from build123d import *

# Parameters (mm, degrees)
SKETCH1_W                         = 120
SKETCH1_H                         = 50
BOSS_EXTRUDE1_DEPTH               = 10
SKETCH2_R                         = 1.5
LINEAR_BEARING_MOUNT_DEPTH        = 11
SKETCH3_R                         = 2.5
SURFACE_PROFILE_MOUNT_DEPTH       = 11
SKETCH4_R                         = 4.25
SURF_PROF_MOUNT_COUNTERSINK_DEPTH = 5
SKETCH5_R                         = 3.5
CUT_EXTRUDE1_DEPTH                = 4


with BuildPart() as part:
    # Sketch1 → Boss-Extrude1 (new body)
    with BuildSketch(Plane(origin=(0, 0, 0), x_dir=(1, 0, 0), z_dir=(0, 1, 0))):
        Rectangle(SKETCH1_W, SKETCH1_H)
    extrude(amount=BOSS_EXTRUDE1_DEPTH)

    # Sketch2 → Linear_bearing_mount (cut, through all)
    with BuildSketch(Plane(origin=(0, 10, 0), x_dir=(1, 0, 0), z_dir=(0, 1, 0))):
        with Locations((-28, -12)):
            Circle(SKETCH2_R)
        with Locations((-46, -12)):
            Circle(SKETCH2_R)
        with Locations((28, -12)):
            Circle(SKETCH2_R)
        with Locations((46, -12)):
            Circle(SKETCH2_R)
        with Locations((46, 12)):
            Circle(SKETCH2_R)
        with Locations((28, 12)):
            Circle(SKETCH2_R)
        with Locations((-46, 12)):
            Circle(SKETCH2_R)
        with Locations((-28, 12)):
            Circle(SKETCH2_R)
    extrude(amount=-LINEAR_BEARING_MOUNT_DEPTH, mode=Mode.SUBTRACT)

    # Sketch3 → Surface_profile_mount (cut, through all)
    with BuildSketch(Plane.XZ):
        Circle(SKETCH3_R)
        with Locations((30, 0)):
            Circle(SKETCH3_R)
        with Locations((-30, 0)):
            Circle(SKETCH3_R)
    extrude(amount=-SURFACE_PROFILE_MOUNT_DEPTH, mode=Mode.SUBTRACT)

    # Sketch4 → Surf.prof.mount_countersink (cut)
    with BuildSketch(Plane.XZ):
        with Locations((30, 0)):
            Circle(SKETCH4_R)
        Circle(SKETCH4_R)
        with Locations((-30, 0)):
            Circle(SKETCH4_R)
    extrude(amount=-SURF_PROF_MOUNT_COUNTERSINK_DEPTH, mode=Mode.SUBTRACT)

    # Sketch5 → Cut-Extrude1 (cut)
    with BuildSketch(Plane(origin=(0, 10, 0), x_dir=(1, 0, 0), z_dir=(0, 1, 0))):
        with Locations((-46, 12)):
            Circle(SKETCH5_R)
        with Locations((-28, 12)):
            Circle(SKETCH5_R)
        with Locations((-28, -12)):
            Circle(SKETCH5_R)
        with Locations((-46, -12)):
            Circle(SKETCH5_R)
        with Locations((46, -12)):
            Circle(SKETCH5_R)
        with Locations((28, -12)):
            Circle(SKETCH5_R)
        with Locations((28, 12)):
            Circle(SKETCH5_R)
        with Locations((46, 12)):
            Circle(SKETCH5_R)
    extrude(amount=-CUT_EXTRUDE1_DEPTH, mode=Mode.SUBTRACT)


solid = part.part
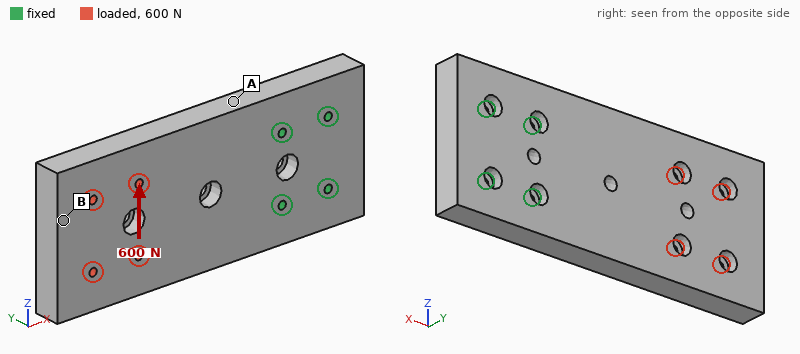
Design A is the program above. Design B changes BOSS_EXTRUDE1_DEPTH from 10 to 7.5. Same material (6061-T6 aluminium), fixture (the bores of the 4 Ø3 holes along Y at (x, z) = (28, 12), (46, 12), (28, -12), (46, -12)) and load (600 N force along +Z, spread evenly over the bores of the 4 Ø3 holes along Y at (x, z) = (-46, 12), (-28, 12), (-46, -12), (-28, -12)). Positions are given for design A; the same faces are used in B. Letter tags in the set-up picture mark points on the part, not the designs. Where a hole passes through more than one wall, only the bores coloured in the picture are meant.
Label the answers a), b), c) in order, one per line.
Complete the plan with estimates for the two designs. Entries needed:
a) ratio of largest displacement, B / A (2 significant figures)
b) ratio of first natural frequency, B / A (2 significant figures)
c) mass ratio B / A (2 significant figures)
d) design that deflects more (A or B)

a) 1.2
b) 0.79
c) 0.75
d) B
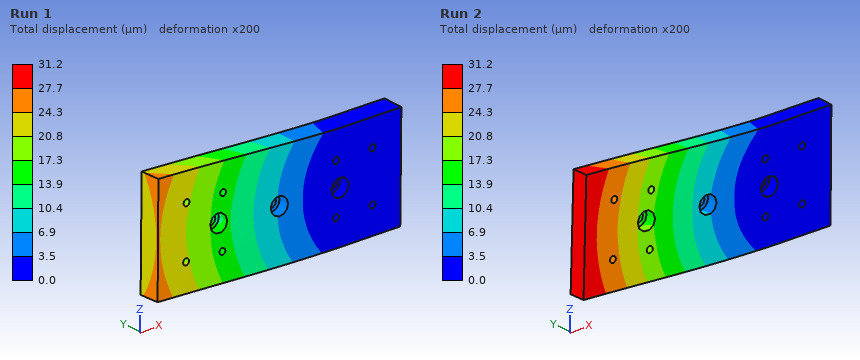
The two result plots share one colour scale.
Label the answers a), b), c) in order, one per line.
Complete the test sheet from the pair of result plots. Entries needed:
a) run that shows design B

a) Run 2
